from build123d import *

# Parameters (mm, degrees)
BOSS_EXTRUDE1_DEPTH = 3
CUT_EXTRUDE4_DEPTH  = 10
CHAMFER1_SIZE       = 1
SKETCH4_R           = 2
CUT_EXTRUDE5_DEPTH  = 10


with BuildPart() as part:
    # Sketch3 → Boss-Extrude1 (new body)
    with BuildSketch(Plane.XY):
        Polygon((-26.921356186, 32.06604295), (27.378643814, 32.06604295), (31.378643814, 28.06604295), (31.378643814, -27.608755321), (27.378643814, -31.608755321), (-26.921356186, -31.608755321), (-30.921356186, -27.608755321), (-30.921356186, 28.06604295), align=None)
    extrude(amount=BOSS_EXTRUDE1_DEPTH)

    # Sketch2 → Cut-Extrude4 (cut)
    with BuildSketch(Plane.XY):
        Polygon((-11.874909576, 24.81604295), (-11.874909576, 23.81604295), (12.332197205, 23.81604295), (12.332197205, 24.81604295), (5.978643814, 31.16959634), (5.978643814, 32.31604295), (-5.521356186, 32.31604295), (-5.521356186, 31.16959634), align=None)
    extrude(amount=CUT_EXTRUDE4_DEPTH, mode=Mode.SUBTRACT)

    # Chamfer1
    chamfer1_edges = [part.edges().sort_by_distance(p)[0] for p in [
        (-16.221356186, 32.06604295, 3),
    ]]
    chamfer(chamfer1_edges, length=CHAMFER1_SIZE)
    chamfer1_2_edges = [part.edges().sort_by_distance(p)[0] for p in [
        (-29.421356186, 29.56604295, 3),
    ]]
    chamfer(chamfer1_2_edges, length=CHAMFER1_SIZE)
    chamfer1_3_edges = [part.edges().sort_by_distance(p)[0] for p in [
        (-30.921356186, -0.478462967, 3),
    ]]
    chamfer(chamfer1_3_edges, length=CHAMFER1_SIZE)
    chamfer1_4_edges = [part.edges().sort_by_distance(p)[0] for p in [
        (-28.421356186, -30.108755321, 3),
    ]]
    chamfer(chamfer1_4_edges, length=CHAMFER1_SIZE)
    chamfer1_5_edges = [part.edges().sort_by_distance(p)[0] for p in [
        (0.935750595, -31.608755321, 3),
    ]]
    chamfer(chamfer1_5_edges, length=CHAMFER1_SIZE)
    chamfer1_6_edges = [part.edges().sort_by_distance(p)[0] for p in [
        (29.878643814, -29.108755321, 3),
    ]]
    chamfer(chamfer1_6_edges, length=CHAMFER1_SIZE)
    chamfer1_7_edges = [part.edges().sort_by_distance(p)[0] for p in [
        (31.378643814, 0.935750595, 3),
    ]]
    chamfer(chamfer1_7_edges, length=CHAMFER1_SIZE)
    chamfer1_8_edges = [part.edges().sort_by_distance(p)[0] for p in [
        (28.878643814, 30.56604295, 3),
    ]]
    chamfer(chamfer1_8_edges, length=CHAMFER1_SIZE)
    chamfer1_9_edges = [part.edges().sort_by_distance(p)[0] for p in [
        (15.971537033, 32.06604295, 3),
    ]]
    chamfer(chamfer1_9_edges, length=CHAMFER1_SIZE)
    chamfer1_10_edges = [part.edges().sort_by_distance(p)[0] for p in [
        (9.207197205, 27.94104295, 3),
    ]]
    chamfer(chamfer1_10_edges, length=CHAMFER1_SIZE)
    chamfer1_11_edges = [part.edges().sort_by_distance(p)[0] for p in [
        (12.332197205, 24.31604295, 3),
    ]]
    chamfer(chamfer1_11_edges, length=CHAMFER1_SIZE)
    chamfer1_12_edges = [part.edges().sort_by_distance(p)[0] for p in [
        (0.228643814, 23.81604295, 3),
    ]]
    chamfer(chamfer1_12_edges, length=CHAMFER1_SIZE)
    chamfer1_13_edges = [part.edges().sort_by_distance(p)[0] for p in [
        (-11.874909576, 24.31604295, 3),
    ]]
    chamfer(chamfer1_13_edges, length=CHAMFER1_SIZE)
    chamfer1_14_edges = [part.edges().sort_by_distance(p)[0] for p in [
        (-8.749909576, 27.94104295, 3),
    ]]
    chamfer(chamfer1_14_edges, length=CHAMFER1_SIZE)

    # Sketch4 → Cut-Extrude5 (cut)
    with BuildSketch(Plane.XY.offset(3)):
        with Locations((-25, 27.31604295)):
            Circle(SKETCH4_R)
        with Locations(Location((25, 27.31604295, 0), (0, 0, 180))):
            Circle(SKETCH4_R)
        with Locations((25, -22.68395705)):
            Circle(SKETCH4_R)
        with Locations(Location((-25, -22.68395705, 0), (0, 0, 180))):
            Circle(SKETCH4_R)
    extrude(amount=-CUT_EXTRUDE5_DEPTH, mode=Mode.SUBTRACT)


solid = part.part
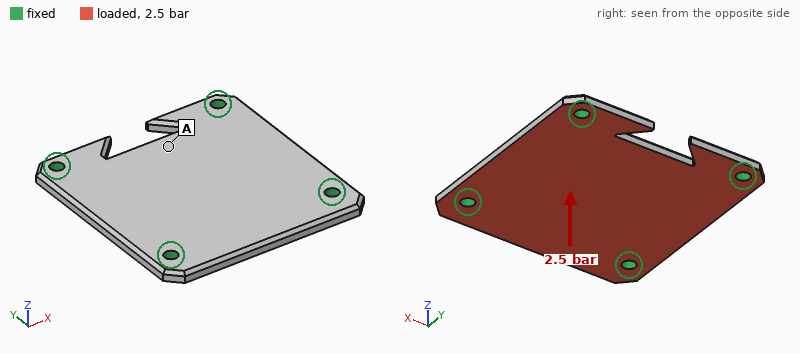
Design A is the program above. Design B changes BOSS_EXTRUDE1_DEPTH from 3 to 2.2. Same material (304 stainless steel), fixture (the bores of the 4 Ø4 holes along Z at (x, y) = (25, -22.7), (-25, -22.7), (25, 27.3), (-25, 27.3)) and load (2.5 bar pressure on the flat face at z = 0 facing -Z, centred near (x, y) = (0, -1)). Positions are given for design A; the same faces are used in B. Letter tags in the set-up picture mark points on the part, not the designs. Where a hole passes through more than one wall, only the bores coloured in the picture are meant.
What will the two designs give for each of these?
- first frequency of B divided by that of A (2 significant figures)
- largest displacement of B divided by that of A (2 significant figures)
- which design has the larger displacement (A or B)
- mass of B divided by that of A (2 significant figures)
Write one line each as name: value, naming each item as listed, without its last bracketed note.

first frequency of B divided by that of A: 0.75
largest displacement of B divided by that of A: 2.4
which design has the larger displacement: B
mass of B divided by that of A: 0.73
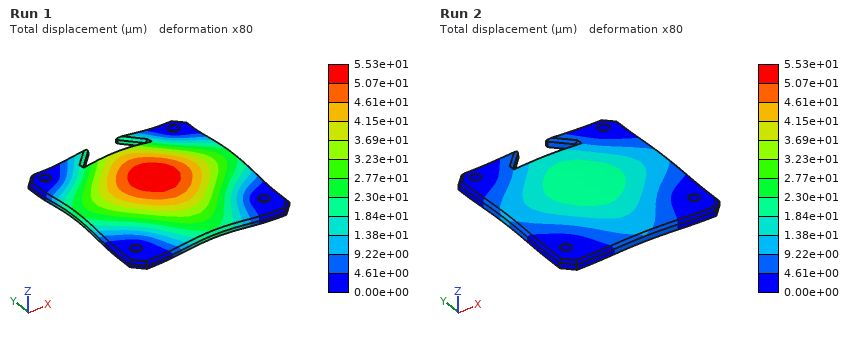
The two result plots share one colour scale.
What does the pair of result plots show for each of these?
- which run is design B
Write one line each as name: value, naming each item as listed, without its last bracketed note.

which run is design B: Run 1
